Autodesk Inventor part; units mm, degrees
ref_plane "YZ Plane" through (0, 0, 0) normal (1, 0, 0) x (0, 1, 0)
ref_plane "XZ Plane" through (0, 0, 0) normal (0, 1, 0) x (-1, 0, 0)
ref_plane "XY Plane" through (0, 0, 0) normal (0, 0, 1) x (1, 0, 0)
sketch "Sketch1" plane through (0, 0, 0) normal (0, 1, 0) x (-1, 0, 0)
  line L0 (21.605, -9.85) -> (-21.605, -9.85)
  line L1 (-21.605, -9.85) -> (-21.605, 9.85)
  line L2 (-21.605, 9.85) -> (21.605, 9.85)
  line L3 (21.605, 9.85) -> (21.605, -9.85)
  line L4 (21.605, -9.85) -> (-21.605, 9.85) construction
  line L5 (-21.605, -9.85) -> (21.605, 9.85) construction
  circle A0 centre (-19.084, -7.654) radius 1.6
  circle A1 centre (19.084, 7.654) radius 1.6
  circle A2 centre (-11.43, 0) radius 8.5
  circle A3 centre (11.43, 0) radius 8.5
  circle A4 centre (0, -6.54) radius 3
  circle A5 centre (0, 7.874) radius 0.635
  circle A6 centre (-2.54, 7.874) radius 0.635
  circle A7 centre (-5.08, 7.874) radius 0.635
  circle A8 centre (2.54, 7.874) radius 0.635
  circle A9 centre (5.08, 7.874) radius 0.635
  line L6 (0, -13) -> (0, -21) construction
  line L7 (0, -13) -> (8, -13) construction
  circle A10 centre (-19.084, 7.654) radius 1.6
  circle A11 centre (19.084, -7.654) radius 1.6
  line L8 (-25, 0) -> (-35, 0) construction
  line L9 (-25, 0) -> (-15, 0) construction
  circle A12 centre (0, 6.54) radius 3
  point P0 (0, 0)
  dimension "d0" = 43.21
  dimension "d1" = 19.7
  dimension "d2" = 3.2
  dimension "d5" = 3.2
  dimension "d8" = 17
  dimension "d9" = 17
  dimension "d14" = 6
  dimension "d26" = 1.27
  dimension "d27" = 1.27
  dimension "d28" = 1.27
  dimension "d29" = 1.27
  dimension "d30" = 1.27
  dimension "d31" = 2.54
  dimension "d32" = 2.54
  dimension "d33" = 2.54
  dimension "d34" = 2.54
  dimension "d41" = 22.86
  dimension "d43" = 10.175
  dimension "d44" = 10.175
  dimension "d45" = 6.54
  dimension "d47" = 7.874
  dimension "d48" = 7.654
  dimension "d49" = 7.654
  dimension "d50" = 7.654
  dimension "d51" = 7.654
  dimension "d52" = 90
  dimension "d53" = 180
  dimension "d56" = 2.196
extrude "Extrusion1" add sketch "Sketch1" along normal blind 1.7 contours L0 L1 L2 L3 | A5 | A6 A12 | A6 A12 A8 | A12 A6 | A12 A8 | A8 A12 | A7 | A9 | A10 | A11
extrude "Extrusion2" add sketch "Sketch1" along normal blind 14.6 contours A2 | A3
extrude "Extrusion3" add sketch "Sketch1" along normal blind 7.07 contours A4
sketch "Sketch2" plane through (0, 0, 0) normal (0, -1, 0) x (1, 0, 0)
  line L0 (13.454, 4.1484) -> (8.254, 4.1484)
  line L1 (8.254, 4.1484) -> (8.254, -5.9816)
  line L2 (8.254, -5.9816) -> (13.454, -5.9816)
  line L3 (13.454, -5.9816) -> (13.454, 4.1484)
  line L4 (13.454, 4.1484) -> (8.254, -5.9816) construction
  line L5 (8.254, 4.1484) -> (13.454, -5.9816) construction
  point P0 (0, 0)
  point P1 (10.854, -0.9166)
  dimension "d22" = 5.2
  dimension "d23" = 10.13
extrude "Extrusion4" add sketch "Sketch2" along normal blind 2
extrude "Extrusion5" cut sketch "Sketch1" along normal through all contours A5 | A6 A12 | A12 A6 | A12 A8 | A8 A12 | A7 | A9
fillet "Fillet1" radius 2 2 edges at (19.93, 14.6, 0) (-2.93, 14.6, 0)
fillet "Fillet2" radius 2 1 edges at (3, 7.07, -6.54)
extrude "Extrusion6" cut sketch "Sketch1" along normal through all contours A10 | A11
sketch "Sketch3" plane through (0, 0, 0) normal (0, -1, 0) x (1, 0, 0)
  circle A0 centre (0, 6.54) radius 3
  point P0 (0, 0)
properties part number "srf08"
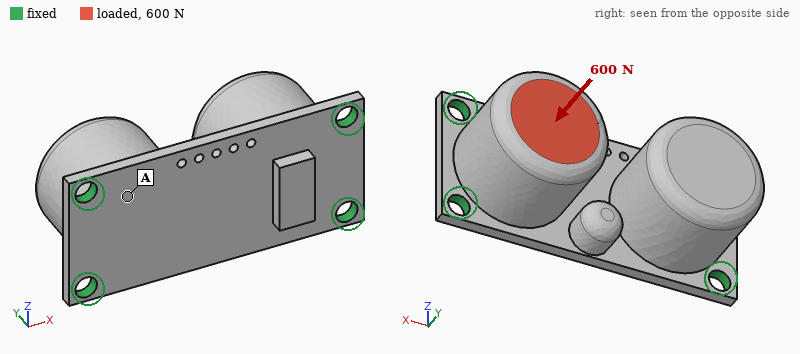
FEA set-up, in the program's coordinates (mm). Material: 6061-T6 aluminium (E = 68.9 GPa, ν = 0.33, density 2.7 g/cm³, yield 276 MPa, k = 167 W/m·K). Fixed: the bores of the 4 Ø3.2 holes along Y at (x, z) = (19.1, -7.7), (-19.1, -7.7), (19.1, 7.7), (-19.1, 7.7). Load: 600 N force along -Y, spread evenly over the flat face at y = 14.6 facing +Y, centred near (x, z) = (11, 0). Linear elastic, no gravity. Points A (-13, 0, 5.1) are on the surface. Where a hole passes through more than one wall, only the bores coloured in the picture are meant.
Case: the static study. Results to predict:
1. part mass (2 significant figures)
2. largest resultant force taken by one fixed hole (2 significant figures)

20 g
260 N
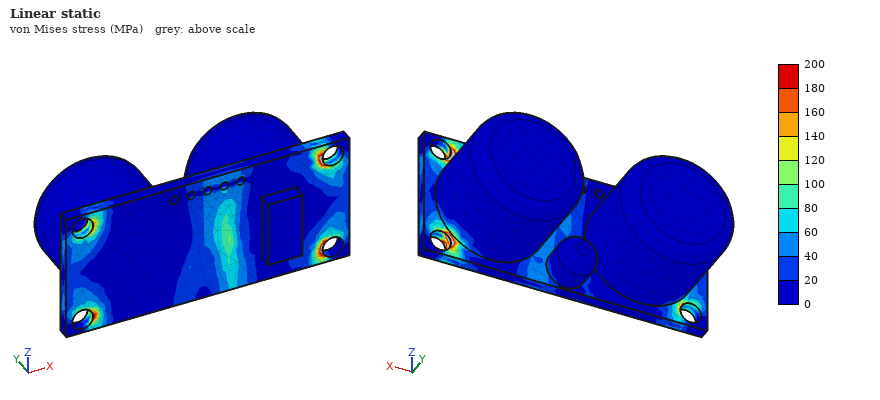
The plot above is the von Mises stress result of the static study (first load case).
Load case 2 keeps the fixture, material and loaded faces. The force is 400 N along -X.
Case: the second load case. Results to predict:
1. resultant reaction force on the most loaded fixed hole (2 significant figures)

190 N
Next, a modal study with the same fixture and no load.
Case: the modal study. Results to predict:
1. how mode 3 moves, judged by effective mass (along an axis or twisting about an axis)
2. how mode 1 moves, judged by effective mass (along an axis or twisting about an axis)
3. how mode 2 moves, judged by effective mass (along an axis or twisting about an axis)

along Z
along Y
along X
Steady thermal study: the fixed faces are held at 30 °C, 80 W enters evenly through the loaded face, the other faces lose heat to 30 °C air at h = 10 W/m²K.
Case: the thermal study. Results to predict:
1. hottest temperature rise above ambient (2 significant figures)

77 K
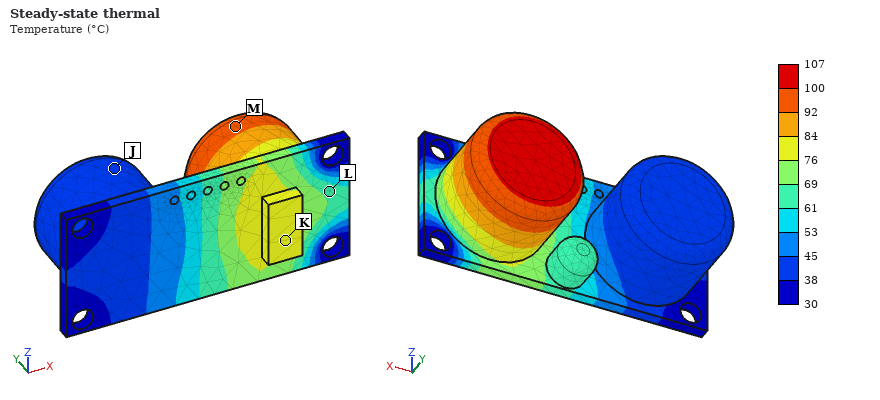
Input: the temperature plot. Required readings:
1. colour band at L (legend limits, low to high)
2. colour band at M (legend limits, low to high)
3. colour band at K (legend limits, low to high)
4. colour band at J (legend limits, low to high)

61 to 69 °C
92 to 100 °C
76 to 84 °C
38 to 45 °C
